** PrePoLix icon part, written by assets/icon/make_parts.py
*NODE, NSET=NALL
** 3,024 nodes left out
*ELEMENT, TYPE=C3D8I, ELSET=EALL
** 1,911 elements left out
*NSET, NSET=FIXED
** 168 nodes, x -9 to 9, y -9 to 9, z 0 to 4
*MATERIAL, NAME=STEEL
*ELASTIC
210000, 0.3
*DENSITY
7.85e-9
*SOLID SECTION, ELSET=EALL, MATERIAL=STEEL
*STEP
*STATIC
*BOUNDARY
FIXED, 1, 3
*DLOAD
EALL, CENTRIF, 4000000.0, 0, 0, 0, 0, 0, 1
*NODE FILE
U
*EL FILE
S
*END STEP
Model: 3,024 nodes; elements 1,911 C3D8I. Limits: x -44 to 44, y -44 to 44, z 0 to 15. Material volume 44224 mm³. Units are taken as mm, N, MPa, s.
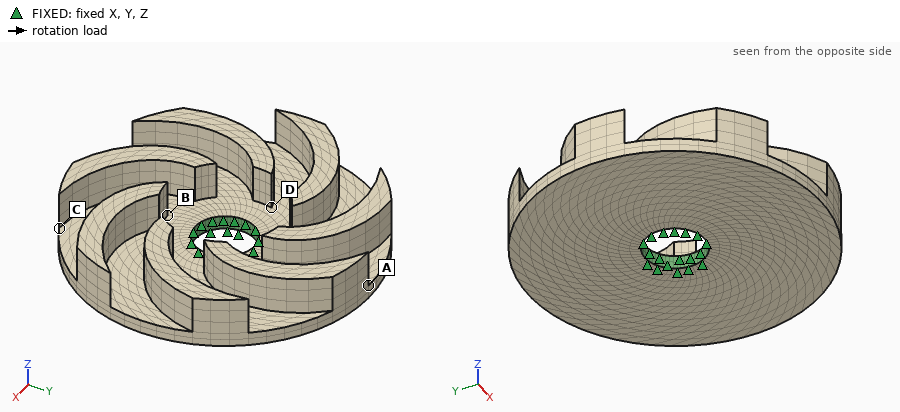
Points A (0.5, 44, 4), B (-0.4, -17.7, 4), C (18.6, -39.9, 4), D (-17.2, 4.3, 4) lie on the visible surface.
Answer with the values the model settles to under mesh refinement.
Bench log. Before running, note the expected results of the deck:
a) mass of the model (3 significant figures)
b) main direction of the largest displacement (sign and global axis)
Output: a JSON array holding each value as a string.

["0.347 kg", "-Z"]
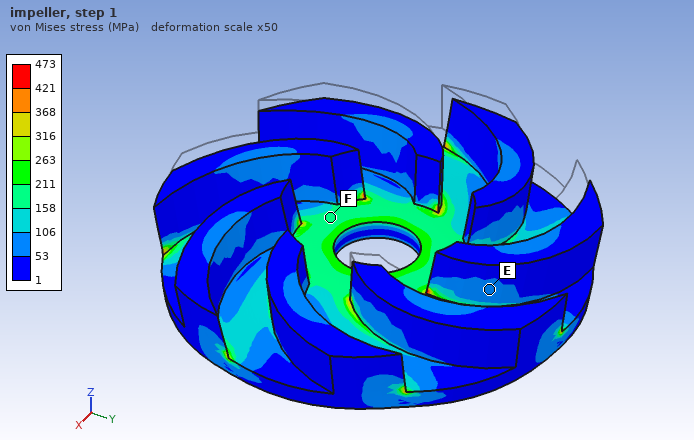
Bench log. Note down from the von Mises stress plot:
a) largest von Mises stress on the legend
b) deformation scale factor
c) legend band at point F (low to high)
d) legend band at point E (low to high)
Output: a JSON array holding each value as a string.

["473 MPa", "50", "158 to 211 MPa", "53 to 106 MPa"]
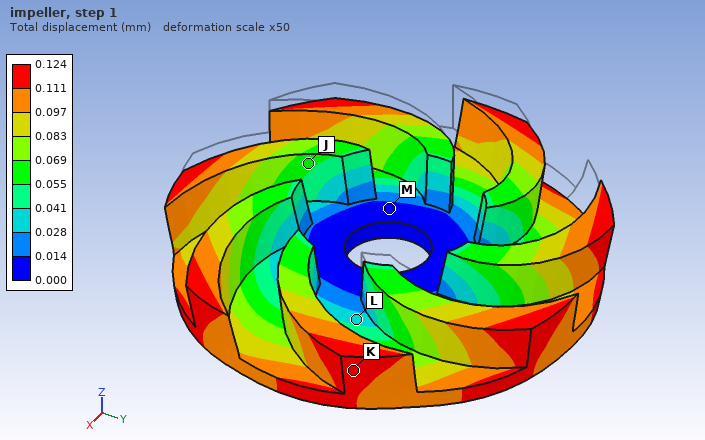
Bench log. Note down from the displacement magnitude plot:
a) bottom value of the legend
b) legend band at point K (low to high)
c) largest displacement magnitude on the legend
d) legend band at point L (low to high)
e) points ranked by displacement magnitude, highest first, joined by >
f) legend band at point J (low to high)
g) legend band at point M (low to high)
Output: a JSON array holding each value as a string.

["0.000 mm", "0.111 to 0.124 mm", "0.124 mm", "0.028 to 0.041 mm", "K > J > L > M", "0.055 to 0.069 mm", "0.000 to 0.014 mm"]
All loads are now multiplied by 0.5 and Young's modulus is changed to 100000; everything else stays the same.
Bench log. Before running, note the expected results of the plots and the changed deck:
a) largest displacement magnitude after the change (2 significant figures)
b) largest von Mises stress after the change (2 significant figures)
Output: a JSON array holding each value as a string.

["0.13 mm", "240 MPa"]
